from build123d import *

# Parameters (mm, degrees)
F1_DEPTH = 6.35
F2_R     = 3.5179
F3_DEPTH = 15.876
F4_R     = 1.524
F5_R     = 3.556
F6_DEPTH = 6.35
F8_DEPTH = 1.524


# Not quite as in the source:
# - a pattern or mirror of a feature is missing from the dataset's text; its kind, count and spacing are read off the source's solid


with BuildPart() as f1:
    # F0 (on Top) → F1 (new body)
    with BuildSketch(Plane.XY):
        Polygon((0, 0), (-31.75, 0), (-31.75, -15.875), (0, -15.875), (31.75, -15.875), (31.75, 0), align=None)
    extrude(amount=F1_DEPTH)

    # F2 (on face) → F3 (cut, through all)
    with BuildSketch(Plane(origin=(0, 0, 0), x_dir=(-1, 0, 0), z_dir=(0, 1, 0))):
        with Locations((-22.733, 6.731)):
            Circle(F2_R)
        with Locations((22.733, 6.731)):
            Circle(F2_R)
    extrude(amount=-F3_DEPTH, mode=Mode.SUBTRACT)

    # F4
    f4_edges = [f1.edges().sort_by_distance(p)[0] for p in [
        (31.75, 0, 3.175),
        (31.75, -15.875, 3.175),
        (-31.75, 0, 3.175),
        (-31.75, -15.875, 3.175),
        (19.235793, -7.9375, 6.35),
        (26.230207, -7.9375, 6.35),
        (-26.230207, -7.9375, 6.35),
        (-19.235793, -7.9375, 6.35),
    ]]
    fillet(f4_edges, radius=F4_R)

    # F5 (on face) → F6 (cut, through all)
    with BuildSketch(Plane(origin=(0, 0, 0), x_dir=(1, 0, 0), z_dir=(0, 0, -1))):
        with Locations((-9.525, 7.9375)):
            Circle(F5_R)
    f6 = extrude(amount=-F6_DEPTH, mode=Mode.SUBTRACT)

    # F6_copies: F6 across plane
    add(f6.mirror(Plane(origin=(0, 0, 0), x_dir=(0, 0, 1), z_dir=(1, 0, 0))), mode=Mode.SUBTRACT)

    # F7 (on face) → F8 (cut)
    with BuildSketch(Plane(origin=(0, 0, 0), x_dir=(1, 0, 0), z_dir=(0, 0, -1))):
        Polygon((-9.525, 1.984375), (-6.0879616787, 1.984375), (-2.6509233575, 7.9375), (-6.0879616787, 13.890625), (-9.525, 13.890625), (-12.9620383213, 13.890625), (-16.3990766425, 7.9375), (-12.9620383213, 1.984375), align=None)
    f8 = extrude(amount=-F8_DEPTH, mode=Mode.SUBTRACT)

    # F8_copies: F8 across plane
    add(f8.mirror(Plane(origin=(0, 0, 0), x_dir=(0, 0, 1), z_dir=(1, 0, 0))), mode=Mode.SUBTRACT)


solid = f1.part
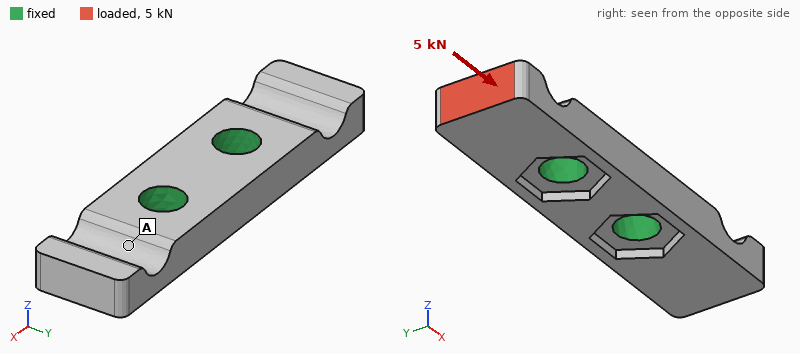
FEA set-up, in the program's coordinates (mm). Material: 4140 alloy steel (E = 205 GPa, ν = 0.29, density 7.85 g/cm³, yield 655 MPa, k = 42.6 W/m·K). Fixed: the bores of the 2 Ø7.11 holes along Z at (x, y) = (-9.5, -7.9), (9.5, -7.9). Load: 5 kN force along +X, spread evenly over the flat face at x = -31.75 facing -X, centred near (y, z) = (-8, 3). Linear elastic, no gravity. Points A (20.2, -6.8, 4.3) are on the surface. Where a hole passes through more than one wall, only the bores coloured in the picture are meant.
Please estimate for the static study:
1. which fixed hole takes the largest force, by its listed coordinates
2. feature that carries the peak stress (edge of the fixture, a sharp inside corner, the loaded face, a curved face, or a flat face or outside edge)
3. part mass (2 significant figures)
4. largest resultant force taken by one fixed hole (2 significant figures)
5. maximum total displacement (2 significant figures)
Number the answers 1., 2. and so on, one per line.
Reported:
1. (-9.5, -7.9)
2. a curved face
3. 40 g
4. 4.6 kN
5. 42 µm
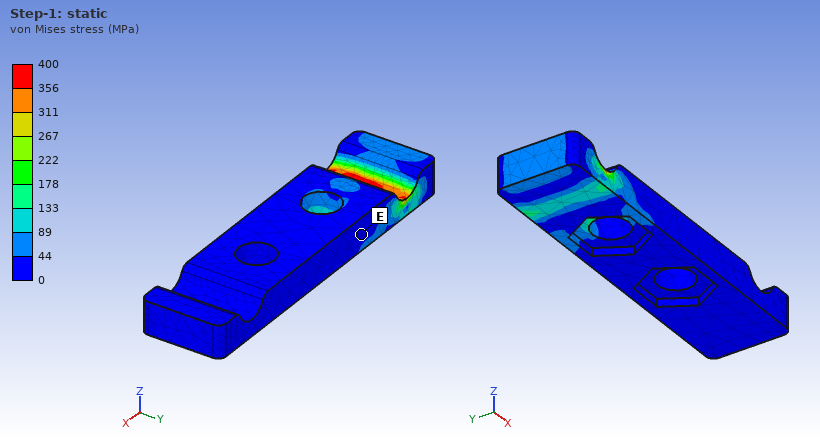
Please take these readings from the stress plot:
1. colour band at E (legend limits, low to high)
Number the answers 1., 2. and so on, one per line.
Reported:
1. 0 to 44 MPa
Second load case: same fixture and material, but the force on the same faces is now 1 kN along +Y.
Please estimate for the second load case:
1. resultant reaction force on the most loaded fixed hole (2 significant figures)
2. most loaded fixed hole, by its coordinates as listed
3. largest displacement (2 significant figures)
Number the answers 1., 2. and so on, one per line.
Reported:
1. 1.3 kN
2. (-9.5, -7.9)
3. 21 µm
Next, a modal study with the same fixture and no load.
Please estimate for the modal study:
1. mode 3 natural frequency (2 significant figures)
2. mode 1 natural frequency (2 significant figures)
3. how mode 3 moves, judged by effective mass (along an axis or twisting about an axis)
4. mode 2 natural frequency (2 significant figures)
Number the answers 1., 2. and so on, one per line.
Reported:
1. 17 kHz
2. 8700 Hz
3. twisting about Z
4. 8800 Hz
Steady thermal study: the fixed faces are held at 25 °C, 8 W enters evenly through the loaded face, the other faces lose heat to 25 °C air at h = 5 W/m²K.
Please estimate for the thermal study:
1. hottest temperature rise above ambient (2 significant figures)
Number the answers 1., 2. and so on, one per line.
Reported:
1. 53 K
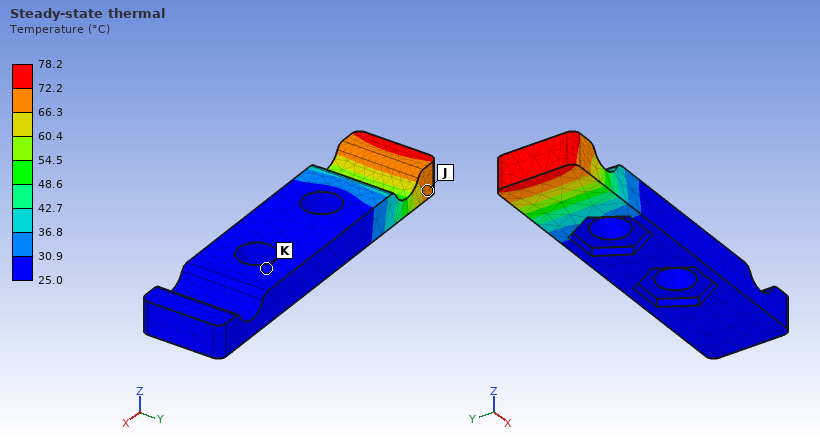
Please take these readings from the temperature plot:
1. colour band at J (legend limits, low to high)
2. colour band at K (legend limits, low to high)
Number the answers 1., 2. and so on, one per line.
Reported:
1. 66.3 to 72.2 °C
2. 25.0 to 30.9 °C
